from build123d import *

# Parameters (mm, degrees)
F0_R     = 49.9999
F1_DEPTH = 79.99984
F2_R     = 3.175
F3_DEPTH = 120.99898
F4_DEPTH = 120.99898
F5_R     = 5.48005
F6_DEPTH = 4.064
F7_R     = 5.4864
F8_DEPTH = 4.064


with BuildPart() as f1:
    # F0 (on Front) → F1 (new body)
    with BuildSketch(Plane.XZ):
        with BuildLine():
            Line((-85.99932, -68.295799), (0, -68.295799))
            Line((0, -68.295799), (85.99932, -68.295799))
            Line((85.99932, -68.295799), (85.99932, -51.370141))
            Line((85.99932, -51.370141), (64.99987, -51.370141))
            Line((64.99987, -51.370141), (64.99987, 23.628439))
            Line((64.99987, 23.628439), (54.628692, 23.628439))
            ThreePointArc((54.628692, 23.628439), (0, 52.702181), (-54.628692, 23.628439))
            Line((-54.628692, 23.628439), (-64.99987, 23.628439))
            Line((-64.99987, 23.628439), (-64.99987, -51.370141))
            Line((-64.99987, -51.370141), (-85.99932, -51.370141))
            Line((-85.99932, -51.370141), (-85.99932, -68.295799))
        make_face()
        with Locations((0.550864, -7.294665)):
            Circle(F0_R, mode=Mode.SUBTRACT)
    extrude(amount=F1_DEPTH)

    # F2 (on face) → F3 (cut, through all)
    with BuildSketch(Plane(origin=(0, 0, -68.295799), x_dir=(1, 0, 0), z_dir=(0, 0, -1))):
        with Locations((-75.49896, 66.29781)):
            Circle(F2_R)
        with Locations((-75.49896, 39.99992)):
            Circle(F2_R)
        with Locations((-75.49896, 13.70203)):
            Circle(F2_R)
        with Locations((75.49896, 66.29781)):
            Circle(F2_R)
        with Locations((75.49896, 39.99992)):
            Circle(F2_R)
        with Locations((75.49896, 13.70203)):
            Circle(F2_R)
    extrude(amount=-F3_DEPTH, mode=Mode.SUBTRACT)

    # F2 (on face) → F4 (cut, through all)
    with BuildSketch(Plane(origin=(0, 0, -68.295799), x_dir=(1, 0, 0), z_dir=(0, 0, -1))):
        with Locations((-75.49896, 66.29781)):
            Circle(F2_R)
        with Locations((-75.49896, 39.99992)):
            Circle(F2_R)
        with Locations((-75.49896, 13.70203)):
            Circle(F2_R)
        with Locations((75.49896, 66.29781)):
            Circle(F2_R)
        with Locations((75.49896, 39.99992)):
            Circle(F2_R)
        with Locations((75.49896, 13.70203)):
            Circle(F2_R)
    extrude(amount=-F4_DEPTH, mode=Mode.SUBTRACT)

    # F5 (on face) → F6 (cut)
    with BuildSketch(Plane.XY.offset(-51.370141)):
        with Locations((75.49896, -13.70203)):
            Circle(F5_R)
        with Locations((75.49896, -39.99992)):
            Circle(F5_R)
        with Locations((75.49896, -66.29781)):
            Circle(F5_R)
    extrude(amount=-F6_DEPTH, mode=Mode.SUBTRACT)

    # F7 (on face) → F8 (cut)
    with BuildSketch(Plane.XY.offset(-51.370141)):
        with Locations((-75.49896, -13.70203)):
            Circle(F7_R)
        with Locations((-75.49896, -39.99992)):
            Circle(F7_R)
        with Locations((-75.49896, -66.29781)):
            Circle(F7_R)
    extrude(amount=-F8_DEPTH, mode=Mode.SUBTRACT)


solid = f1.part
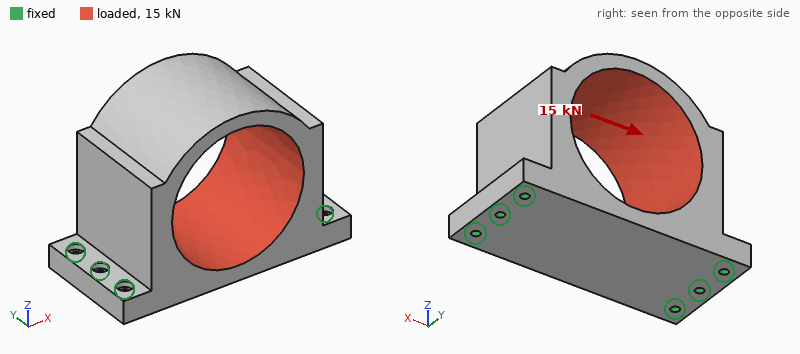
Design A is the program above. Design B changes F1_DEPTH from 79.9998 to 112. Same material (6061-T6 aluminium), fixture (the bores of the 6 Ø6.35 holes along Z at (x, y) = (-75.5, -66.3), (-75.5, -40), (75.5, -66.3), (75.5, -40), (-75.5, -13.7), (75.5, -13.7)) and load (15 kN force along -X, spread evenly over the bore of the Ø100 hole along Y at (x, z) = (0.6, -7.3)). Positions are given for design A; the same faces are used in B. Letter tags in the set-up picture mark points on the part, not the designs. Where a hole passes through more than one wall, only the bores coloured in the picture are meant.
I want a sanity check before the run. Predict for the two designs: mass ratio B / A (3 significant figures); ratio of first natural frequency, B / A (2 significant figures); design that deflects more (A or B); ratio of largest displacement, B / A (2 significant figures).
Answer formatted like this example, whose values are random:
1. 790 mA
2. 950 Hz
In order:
1. 1.40
2. 0.90
3. A
4. 0.76
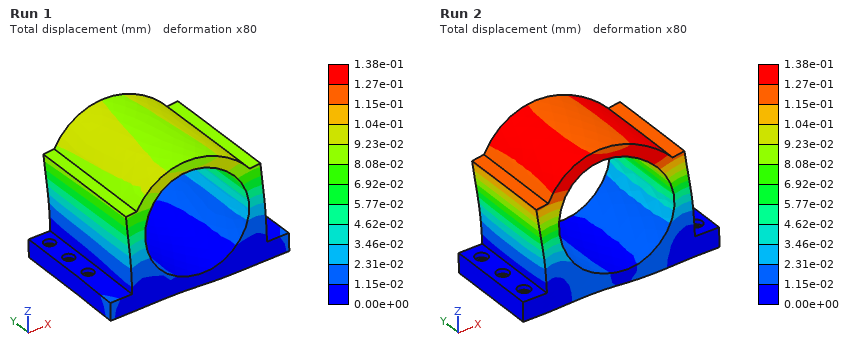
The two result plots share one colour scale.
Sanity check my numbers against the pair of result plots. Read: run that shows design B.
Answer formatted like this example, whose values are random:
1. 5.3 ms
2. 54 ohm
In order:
1. Run 1
